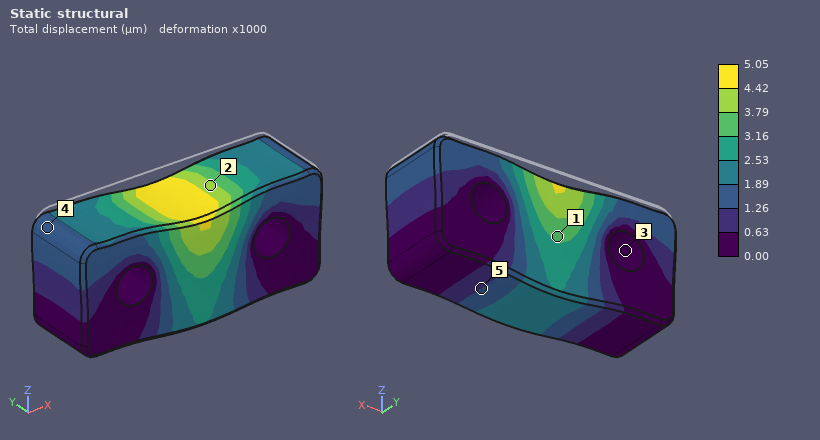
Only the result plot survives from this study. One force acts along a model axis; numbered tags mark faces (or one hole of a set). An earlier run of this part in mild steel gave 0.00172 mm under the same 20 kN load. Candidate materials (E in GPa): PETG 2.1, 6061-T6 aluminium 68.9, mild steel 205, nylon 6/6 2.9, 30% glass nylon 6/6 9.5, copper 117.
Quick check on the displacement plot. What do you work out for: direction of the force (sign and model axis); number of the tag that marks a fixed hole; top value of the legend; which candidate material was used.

-Z
3
5.05 µm
6061-T6 aluminium
